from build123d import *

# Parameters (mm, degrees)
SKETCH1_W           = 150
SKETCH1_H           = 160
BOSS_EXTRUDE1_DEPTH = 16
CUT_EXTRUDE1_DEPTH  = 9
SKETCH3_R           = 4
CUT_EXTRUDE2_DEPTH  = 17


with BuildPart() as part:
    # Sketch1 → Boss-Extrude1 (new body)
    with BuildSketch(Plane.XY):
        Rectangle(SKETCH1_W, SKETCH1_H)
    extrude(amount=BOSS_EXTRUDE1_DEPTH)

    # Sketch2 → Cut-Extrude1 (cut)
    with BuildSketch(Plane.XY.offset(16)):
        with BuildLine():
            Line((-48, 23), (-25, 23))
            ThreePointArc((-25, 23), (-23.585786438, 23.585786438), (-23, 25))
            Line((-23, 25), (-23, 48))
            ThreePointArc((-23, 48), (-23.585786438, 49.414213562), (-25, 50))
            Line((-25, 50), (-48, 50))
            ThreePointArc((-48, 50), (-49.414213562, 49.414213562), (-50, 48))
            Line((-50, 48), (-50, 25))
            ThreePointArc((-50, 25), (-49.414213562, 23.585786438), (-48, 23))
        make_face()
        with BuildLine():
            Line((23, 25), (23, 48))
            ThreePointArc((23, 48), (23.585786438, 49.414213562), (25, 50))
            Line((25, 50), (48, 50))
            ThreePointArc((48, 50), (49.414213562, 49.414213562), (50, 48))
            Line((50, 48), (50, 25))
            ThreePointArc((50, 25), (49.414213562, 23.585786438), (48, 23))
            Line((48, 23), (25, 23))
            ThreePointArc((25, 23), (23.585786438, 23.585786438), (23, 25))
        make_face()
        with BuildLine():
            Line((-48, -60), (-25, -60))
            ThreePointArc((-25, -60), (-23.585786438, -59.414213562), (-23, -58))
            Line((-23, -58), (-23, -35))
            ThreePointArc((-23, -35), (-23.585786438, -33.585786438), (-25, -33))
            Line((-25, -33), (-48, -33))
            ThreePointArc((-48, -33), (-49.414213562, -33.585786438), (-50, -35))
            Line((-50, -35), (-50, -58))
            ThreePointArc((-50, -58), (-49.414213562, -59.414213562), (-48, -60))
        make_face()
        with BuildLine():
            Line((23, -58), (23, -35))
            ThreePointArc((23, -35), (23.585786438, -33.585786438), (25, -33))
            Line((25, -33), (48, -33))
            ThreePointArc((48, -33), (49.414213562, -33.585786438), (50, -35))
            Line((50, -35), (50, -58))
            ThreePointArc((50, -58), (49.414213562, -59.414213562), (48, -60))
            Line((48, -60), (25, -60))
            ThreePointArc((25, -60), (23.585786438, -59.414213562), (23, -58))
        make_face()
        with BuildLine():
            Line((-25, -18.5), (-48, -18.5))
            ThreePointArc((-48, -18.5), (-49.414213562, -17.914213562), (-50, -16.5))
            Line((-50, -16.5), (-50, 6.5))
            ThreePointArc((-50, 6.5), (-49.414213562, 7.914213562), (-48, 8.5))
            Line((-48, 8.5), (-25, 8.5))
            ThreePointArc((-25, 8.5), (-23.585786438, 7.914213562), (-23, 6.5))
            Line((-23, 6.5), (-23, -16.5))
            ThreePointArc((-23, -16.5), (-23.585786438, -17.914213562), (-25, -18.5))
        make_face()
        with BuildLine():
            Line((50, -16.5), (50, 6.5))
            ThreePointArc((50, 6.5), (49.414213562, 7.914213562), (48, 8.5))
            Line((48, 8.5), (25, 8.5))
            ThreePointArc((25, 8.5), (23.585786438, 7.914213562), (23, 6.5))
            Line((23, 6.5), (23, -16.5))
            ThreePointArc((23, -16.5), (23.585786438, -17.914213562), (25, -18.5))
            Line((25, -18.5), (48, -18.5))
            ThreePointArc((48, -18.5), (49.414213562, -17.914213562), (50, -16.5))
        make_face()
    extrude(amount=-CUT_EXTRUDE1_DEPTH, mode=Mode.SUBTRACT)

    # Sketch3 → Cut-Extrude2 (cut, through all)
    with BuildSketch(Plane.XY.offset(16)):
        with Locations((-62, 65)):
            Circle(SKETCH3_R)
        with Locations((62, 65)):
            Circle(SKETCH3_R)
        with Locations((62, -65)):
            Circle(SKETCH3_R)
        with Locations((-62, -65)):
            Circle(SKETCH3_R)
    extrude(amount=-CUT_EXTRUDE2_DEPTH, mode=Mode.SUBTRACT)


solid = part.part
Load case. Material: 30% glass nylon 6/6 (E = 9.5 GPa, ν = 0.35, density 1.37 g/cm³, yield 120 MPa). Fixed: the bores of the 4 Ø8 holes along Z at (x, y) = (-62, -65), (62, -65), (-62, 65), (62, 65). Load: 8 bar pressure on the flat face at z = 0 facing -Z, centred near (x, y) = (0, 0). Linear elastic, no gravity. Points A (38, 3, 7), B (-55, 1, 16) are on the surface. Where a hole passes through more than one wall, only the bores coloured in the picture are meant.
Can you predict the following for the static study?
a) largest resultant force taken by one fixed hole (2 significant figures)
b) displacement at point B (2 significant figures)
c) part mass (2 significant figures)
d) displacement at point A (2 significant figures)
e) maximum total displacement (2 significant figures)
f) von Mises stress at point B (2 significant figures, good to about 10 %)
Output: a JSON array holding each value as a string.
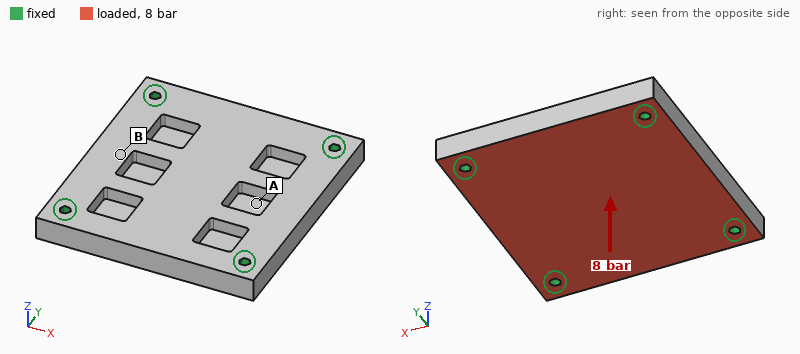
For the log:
["4.9 kN", "0.43 mm", "470 g", "0.56 mm", "0.65 mm", "25 MPa"]
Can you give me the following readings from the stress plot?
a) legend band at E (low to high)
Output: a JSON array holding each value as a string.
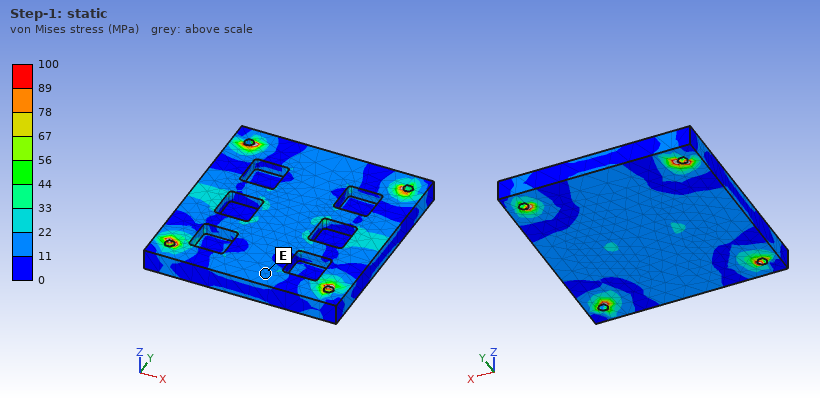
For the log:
["11 to 22 MPa"]
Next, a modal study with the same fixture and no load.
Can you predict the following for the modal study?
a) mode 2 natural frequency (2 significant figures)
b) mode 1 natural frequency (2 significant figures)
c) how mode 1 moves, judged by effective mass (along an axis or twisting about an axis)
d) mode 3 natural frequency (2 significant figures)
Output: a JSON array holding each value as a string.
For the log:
["2500 Hz", "1500 Hz", "along Z", "2500 Hz"]
